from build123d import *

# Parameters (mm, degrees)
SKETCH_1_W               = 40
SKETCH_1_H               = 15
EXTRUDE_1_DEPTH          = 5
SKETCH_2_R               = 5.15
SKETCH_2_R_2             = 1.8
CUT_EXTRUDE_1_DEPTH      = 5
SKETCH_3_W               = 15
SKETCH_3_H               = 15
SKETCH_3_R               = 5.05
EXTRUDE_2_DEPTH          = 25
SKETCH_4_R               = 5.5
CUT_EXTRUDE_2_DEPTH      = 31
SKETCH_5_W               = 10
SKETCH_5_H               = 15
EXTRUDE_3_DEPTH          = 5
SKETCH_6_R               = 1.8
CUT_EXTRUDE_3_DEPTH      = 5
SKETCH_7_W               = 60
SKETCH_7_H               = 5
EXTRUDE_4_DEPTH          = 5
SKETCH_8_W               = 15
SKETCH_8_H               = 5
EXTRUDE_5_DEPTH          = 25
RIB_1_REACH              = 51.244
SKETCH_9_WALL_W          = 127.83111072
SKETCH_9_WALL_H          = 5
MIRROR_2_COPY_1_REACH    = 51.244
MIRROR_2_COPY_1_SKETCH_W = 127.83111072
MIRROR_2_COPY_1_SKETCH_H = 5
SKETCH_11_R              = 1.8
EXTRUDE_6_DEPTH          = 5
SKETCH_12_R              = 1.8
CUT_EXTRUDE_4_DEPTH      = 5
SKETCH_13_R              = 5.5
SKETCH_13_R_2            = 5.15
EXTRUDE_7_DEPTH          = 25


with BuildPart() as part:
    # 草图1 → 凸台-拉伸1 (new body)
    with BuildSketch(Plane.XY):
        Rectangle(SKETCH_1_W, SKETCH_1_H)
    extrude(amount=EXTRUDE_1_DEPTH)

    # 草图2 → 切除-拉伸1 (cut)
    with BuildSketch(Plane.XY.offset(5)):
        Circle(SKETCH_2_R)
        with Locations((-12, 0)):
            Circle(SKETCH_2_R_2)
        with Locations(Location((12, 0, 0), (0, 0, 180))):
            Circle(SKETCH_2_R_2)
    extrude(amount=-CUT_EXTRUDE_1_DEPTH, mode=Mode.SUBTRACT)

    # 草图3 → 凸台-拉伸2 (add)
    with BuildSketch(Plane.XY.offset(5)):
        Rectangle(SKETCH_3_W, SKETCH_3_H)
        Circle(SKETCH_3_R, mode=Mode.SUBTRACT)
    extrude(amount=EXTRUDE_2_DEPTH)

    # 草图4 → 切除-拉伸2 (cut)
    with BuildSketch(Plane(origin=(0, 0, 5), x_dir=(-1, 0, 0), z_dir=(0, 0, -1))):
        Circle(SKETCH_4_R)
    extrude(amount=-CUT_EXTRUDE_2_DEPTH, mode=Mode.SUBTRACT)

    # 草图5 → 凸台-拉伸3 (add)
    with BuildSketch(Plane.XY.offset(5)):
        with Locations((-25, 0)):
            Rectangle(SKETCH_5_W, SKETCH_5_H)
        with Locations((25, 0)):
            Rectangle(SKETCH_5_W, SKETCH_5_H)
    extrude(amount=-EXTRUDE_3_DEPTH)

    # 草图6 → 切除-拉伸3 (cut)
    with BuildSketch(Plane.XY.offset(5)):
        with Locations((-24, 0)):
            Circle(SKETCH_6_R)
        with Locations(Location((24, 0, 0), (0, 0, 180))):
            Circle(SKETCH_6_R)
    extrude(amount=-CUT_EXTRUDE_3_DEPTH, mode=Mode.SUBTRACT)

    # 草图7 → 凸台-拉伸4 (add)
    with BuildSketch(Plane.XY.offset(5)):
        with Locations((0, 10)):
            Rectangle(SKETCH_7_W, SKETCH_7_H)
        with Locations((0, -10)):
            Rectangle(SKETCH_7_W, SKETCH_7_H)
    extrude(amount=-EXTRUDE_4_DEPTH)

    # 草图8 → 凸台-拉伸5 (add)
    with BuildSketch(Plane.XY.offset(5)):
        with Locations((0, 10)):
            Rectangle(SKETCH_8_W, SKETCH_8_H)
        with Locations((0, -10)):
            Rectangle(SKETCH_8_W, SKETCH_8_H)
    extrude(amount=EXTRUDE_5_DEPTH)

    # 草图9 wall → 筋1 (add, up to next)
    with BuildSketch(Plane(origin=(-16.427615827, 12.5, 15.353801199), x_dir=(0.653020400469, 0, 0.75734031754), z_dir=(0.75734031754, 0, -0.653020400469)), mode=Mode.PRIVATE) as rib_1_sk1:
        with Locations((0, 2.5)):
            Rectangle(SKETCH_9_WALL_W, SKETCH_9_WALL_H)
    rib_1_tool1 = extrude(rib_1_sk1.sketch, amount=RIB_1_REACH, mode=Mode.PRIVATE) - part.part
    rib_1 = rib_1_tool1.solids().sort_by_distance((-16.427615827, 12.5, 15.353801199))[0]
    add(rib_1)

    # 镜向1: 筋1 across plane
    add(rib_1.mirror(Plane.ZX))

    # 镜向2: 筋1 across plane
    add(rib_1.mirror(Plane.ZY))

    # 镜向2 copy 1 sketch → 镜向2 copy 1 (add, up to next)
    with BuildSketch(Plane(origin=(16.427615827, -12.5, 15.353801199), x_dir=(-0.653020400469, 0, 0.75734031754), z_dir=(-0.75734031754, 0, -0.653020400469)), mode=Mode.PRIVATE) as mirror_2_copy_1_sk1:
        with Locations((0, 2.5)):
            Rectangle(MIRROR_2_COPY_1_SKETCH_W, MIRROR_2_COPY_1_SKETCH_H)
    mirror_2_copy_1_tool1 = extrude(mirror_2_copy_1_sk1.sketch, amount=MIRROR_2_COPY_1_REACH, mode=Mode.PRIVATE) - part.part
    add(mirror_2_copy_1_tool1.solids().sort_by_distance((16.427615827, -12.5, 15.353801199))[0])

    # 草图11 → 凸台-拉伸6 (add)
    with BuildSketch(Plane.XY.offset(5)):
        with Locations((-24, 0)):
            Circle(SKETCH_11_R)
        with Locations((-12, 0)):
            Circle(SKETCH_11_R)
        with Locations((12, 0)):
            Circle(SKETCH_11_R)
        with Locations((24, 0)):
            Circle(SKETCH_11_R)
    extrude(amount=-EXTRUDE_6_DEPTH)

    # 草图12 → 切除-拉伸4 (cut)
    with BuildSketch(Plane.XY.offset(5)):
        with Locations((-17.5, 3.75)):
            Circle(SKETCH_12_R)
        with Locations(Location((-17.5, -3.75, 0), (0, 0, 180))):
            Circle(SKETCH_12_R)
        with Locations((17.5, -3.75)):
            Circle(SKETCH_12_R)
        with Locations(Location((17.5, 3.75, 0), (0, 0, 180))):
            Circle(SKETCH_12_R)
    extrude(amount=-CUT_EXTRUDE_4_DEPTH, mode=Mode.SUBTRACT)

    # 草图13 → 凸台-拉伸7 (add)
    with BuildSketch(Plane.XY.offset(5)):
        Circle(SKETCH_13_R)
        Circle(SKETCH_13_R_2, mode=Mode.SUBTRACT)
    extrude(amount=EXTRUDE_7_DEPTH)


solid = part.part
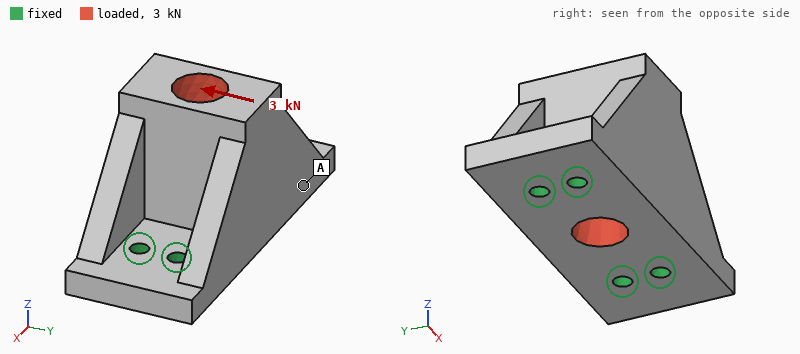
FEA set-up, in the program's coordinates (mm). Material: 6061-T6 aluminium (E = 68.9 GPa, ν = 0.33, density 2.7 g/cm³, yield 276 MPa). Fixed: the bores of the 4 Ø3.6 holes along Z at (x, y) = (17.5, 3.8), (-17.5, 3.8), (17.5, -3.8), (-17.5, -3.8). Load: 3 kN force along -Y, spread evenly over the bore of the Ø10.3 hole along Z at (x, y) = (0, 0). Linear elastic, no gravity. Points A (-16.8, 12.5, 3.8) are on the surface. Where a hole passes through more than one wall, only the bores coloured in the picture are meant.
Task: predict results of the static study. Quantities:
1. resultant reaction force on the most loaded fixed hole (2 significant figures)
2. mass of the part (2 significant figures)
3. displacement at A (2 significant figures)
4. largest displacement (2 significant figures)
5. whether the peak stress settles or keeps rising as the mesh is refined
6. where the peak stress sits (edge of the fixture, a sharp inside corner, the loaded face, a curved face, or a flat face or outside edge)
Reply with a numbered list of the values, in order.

1. 1.6 kN
2. 48 g
3. 16 µm
4. 64 µm
5. keeps rising
6. edge of the fixture
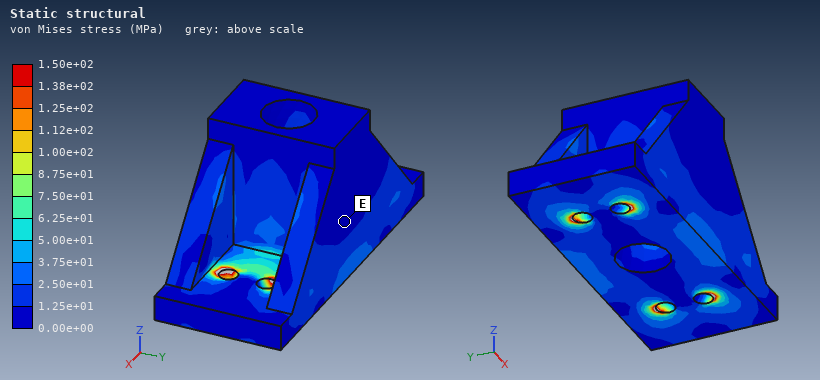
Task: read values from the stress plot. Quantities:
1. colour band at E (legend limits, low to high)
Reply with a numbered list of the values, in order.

1. 0.00e+00 to 1.25e+01 MPa
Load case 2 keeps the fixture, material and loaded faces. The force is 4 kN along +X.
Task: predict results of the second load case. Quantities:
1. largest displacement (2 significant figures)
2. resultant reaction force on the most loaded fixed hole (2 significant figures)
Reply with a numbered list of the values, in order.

1. 18 µm
2. 1.2 kN
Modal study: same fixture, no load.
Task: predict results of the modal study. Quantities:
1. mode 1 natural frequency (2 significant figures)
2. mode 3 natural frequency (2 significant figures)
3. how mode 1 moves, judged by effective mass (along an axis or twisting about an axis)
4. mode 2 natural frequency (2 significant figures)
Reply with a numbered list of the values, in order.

1. 7300 Hz
2. 17 kHz
3. along Y
4. 17 kHz
